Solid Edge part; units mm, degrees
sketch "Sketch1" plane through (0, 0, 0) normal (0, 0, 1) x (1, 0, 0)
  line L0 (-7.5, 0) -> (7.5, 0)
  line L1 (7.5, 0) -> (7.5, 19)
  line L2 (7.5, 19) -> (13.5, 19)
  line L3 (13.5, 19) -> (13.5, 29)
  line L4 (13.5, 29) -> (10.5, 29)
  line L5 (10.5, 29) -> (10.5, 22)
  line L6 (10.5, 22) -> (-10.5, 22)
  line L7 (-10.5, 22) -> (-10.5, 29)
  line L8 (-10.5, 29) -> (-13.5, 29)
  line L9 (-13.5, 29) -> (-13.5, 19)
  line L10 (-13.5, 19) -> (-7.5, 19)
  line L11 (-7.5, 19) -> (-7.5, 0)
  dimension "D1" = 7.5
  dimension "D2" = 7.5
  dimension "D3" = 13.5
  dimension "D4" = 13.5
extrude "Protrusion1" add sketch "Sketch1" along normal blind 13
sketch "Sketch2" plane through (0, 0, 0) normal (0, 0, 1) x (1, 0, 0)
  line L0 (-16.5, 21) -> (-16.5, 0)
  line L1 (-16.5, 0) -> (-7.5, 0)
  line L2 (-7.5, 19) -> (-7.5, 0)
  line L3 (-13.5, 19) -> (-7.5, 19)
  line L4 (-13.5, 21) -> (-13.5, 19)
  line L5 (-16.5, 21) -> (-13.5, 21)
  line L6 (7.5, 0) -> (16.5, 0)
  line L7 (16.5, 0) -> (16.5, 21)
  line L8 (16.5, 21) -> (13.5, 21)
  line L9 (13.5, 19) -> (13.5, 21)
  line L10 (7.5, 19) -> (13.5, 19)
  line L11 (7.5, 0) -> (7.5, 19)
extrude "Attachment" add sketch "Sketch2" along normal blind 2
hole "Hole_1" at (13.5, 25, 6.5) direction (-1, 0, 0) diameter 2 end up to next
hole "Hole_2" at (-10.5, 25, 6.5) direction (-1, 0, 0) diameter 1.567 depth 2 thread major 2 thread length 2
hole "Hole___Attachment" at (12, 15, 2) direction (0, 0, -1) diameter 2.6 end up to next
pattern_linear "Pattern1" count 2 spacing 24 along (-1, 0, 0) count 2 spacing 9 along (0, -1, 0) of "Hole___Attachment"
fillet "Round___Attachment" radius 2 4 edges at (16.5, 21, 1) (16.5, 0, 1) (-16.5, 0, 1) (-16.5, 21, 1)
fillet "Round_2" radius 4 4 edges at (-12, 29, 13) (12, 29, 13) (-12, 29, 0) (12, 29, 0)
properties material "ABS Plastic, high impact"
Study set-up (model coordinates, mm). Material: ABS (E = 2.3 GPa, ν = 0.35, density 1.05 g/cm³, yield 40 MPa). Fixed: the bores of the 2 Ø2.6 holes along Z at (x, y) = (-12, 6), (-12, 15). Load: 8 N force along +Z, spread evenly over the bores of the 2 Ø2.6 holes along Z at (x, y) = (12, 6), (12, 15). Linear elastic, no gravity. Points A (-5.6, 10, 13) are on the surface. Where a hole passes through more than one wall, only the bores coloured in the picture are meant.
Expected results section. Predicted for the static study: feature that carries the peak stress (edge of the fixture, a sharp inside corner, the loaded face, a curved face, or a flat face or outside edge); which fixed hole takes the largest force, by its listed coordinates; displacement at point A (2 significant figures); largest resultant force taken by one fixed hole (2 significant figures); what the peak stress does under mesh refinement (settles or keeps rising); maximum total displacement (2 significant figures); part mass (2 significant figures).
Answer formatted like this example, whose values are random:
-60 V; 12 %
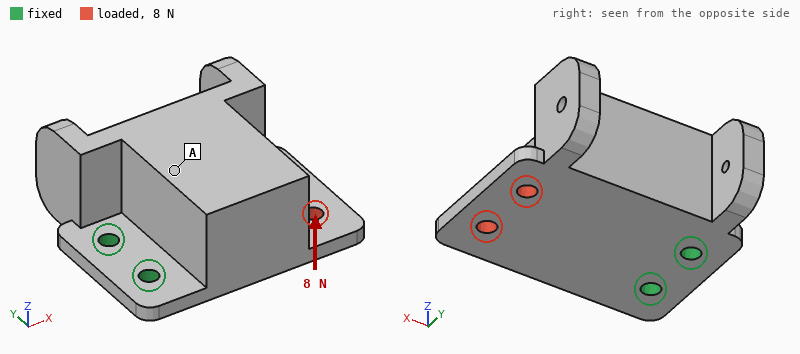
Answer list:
edge of the fixture; (-12, 15); 0.20 mm; 5.4 N; keeps rising; 0.45 mm; 6.2 g
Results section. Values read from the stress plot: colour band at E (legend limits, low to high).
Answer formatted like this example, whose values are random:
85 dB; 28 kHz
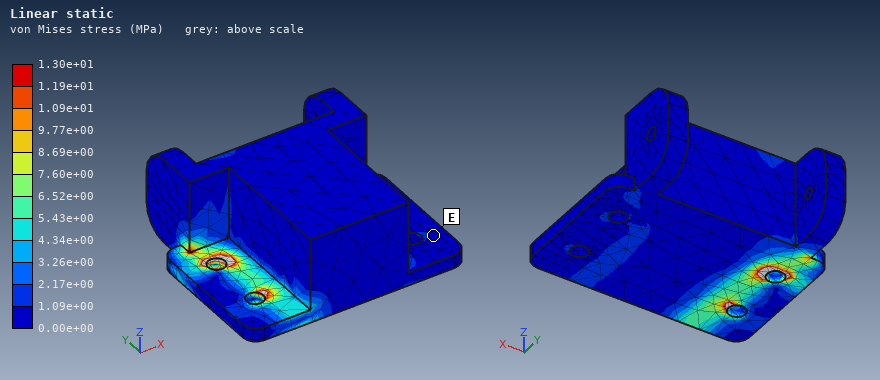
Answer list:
0.00e+00 to 1.09e+00 MPa
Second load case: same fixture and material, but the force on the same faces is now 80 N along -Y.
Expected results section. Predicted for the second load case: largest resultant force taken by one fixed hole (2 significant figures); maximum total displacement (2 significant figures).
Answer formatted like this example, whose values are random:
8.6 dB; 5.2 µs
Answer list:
180 N; 0.25 mm
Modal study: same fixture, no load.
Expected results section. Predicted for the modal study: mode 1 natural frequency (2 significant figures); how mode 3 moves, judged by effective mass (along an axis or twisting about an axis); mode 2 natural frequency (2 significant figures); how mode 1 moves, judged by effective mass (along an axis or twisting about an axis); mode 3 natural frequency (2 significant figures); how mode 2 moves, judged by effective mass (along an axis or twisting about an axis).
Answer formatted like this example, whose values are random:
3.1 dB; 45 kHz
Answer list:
480 Hz; along Y; 1700 Hz; along Z; 2300 Hz; along Y
